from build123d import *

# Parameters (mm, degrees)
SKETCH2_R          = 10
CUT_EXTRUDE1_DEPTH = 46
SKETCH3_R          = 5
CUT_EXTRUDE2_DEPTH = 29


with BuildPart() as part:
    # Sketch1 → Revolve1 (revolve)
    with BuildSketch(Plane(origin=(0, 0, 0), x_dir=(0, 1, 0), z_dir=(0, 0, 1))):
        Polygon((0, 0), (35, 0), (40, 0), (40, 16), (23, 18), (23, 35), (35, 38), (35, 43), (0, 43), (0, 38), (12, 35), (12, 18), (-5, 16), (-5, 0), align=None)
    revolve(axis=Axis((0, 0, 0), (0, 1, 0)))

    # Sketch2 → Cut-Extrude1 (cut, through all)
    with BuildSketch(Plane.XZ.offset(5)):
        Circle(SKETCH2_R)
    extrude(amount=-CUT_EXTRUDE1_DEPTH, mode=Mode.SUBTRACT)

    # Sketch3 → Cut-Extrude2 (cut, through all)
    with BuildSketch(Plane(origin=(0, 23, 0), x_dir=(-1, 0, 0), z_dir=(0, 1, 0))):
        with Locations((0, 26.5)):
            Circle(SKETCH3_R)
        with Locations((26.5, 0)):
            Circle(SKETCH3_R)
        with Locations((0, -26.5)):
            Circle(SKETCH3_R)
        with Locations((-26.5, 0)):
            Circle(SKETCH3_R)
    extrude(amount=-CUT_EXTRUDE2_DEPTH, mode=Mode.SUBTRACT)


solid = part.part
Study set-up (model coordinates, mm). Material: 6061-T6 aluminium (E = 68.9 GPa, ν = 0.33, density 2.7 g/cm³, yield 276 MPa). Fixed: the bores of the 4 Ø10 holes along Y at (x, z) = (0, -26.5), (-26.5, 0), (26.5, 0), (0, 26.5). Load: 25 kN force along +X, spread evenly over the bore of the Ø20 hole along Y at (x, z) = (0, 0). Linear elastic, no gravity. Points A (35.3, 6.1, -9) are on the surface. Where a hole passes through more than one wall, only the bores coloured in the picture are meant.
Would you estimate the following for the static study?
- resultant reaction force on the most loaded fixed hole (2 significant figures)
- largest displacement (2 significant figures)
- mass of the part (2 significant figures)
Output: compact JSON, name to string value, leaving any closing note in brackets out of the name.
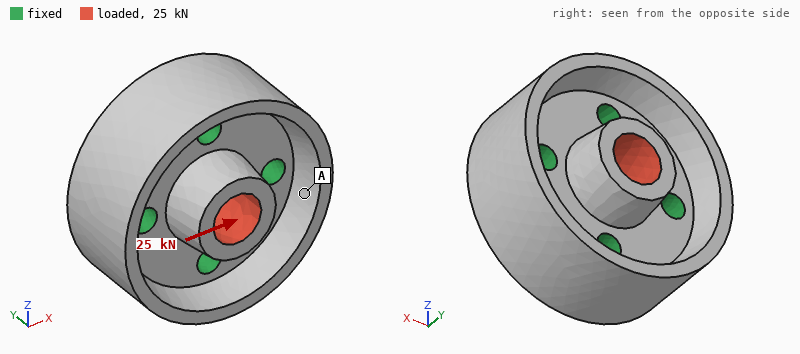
{"resultant reaction force on the most loaded fixed hole": "7.8 kN", "largest displacement": "19 µm", "mass of the part": "310 g"}
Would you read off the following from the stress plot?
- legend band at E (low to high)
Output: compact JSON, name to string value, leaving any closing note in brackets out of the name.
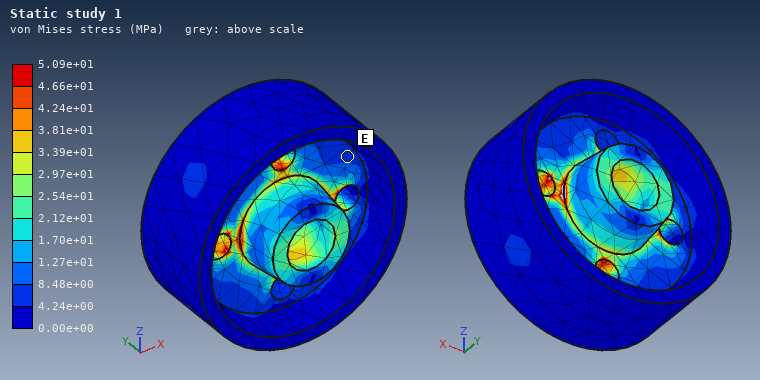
{"legend band at E": "4.24e+00 to 8.48e+00 MPa"}
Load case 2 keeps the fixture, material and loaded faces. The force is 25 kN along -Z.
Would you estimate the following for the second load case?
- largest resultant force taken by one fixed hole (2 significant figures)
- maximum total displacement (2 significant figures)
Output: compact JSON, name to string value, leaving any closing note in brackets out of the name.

{"largest resultant force taken by one fixed hole": "7.8 kN", "maximum total displacement": "19 µm"}
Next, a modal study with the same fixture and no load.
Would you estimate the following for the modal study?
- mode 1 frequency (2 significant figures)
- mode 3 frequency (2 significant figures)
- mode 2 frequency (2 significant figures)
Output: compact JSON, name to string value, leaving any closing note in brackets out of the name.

{"mode 1 frequency": "10 kHz", "mode 3 frequency": "13 kHz", "mode 2 frequency": "13 kHz"}
